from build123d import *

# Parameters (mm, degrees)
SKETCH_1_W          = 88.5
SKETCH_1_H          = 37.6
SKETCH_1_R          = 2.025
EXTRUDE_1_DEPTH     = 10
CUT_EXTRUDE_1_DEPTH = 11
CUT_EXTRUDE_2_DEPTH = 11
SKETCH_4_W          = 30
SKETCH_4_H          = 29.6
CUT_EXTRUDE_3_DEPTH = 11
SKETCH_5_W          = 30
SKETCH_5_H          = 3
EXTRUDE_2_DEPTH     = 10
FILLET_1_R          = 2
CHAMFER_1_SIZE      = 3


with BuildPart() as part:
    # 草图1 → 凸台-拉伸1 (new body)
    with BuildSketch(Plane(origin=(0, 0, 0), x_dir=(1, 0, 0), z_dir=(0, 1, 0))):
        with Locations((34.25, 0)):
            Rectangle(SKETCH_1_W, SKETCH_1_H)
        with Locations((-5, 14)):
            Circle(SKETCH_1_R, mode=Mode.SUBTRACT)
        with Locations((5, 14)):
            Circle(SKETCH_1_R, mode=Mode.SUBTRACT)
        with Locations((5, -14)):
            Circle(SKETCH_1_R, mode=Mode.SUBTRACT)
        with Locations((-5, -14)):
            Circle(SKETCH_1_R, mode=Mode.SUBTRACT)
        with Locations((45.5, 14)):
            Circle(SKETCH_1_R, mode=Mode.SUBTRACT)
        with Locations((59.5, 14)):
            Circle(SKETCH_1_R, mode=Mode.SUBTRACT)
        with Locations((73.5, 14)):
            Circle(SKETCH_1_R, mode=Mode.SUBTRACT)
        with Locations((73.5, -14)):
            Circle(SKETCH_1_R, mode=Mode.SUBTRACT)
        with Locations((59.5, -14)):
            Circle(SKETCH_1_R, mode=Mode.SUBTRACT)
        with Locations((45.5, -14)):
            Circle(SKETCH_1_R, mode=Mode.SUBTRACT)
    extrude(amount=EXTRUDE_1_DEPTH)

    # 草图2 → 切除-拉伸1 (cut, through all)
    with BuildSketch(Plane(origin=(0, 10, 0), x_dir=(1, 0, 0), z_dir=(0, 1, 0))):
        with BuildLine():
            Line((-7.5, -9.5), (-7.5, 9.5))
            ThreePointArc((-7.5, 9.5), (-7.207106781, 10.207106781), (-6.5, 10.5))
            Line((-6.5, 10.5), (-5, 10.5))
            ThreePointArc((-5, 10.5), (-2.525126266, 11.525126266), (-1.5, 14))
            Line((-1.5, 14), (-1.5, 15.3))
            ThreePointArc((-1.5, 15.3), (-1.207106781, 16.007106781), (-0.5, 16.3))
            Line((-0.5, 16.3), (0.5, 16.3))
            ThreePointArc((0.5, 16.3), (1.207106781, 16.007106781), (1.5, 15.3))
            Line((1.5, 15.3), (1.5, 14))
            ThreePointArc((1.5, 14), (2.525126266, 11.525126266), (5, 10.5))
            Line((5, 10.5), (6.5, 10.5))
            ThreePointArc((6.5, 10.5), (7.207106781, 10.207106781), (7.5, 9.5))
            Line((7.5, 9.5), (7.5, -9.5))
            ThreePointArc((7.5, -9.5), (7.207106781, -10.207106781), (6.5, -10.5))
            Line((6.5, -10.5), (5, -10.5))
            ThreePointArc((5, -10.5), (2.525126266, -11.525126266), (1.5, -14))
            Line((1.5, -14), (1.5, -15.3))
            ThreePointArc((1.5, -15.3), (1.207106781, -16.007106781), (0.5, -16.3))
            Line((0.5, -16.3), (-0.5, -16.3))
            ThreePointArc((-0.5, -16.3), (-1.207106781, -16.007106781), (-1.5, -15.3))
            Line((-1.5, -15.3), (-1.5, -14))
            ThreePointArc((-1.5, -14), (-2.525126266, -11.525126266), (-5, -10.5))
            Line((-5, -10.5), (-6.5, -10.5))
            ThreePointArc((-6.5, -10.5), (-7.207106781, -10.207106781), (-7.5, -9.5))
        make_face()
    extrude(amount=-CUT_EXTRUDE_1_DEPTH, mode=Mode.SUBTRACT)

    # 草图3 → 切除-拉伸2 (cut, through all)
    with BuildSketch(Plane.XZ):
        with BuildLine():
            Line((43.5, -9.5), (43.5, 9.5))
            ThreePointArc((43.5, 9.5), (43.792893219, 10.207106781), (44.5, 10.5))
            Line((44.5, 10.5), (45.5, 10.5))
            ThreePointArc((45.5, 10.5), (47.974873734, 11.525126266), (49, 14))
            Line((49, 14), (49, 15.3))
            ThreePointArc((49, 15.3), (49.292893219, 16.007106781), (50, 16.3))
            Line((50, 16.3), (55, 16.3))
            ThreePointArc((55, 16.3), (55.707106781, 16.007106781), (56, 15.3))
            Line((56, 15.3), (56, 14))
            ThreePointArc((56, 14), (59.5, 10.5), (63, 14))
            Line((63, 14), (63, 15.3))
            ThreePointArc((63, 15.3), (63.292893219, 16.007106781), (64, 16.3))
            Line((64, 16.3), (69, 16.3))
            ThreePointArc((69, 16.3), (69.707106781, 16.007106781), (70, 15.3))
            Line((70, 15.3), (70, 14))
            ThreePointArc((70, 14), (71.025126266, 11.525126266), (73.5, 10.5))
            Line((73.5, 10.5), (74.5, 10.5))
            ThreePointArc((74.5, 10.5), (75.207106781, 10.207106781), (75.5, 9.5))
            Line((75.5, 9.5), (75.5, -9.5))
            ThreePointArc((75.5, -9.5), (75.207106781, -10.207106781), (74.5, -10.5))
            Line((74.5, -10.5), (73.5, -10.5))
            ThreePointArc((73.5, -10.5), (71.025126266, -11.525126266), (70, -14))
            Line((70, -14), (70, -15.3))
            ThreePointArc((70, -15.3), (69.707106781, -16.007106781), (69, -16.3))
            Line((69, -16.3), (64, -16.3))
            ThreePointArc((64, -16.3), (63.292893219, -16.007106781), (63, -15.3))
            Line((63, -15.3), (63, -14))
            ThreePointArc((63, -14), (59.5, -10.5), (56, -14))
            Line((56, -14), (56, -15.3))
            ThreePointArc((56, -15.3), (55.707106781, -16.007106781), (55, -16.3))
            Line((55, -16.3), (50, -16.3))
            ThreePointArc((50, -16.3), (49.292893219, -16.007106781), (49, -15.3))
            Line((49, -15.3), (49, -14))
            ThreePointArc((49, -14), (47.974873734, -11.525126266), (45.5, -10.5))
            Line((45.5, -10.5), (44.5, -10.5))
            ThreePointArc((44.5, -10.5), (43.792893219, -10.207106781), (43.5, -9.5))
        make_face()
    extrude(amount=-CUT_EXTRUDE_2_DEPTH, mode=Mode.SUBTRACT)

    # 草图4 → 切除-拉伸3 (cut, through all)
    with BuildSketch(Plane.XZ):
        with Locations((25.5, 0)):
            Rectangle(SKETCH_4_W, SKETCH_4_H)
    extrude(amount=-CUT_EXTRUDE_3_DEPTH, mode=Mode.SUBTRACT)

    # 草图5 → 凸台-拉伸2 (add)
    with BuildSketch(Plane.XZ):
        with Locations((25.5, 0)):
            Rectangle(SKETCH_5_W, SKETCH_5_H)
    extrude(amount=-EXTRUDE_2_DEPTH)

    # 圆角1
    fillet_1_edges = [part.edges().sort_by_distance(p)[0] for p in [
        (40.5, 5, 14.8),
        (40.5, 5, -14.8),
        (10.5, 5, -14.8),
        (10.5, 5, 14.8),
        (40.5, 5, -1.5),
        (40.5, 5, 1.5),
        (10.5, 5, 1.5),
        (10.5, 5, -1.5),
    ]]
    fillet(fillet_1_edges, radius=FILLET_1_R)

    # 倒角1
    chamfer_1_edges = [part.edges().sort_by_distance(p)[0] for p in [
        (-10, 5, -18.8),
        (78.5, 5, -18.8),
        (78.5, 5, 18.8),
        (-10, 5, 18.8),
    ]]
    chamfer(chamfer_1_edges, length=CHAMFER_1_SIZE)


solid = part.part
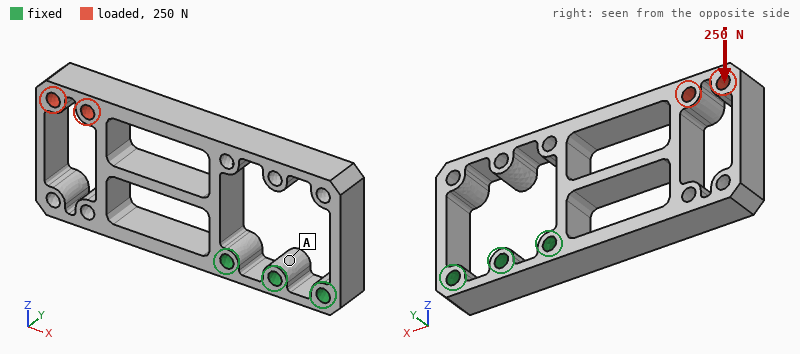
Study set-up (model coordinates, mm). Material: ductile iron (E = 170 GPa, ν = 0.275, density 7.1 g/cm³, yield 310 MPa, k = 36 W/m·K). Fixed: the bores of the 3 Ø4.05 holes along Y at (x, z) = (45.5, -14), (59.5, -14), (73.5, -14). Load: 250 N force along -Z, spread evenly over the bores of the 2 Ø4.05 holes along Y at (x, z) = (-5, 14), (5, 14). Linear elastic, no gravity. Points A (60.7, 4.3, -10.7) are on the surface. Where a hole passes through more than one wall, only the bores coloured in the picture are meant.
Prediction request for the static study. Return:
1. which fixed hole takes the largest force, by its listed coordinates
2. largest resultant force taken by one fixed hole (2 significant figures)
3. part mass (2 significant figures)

(45.5, -14)
370 N
84 g
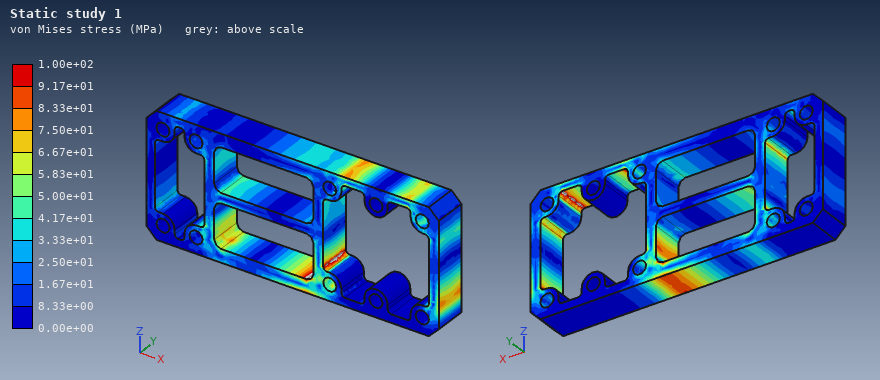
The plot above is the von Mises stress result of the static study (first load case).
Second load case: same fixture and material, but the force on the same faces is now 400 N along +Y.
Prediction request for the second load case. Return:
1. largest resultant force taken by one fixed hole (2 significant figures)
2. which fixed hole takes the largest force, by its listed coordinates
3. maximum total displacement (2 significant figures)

610 N
(45.5, -14)
0.43 mm
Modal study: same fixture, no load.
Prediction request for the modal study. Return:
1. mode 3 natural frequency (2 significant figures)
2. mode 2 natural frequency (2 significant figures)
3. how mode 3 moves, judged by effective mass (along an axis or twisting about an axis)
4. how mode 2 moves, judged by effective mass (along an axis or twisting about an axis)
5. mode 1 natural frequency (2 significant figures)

2800 Hz
1300 Hz
twisting about X
along Y
1200 Hz
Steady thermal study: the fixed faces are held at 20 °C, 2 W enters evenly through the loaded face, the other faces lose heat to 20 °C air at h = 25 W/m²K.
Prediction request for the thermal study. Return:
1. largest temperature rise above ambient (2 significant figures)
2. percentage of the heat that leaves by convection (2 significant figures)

20 K
71 %
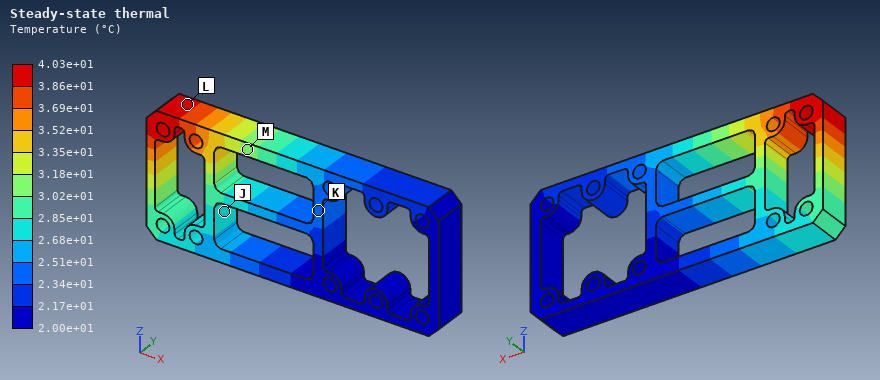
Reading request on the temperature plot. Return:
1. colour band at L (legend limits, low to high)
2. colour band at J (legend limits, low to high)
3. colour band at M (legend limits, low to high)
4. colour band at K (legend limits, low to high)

3.86e+01 to 4.03e+01 °C
2.68e+01 to 2.85e+01 °C
3.02e+01 to 3.18e+01 °C
2.34e+01 to 2.51e+01 °C
